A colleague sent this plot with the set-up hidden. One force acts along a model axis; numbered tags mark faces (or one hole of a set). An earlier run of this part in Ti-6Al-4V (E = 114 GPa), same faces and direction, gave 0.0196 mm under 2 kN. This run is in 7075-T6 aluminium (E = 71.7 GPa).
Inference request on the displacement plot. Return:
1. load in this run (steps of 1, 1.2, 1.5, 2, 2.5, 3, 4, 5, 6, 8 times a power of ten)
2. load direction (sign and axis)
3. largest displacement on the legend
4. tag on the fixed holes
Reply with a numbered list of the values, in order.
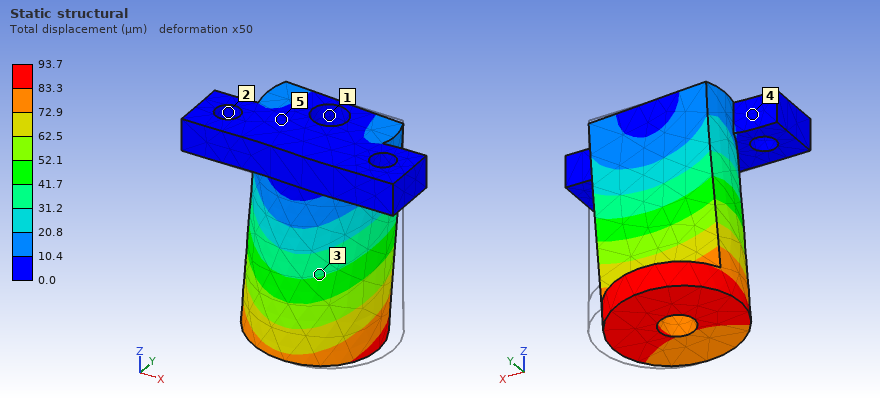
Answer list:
1. 6 kN
2. -X
3. 93.7 µm
4. 2
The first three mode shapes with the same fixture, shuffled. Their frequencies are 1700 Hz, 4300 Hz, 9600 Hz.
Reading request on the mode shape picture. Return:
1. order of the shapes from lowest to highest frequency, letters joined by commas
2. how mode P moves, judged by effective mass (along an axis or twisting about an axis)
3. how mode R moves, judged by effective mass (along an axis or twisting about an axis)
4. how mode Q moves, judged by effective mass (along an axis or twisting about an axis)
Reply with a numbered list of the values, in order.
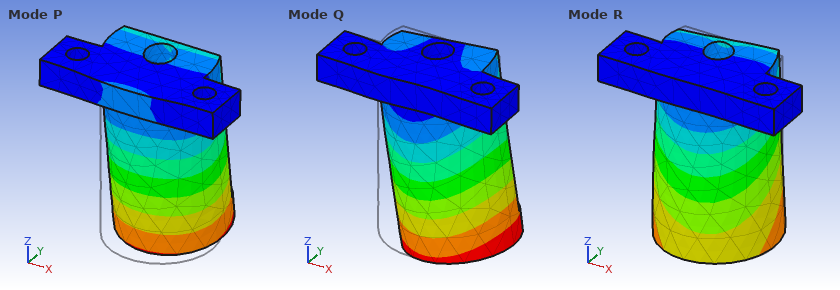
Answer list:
1. P, Q, R
2. along Y
3. twisting about Z
4. along X
